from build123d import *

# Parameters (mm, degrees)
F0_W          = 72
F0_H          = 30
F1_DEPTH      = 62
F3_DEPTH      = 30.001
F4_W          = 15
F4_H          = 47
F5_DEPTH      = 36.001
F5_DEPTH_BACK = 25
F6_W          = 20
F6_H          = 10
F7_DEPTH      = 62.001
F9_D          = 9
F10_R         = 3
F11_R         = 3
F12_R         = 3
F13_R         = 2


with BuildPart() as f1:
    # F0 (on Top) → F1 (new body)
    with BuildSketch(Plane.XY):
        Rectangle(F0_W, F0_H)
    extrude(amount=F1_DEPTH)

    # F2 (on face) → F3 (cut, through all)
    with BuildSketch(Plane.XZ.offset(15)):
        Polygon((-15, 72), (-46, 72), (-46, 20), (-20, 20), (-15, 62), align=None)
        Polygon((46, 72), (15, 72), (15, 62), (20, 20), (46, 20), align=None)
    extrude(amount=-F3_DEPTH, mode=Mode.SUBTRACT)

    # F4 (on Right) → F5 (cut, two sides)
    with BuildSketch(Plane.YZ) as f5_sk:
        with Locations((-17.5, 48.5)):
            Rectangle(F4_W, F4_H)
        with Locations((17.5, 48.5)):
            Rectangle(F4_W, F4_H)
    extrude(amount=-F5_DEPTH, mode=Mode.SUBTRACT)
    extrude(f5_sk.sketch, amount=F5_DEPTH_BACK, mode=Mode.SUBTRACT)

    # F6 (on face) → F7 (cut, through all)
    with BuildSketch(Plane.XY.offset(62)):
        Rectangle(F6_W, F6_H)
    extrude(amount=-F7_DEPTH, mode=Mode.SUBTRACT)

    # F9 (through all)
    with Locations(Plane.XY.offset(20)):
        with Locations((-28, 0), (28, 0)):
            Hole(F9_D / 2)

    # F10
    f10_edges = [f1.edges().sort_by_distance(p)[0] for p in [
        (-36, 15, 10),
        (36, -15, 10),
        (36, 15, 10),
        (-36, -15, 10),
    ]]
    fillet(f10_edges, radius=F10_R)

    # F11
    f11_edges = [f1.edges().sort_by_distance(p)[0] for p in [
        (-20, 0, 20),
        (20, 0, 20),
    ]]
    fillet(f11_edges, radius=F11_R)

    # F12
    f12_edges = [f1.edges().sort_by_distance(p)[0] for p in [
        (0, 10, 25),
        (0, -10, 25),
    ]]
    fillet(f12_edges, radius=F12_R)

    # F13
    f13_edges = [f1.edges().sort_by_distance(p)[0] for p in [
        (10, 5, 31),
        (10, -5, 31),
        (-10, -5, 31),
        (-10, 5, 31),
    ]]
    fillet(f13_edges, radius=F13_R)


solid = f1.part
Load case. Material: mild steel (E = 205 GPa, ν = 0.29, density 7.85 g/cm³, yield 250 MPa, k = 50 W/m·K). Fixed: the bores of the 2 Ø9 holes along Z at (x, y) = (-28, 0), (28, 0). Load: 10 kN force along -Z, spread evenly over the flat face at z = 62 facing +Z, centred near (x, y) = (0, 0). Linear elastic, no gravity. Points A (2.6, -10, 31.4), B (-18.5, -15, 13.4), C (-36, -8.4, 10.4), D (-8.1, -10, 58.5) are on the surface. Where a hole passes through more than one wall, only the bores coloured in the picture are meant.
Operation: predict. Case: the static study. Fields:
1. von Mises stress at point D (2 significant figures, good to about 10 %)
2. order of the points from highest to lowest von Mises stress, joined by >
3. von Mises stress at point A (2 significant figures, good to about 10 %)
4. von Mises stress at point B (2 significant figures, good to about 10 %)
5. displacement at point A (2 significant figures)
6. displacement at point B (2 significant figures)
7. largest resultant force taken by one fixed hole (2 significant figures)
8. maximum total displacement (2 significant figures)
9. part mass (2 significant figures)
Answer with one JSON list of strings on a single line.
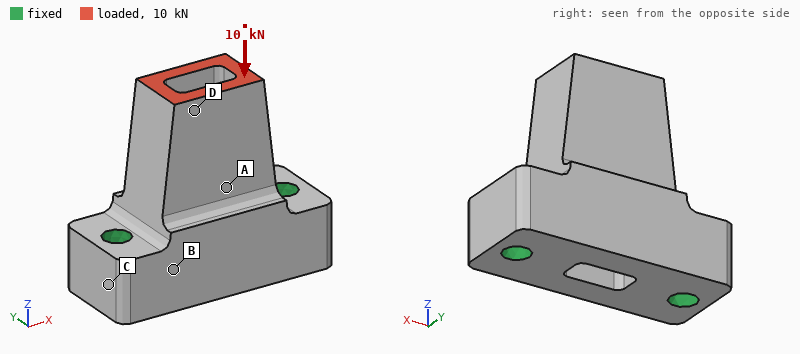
["24 MPa", "D > A > B > C", "17 MPa", "11 MPa", "3.1 µm", "1.5 µm", "5.2 kN", "6.3 µm", "470 g"]
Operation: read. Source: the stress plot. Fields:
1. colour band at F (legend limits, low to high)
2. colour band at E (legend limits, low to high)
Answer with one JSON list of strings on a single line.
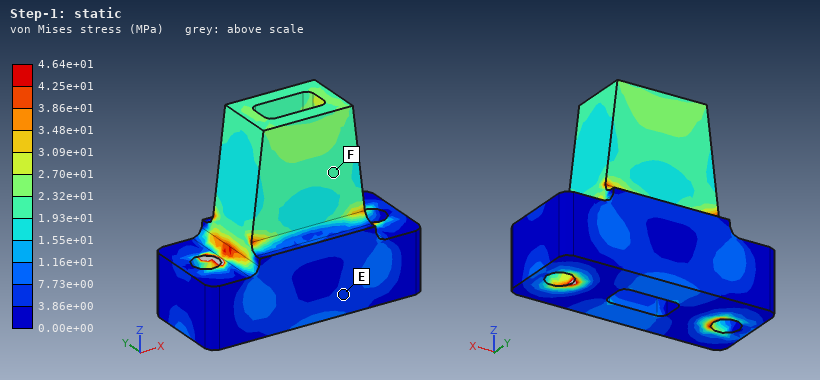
["1.93e+01 to 2.32e+01 MPa", "3.86e+00 to 7.73e+00 MPa"]
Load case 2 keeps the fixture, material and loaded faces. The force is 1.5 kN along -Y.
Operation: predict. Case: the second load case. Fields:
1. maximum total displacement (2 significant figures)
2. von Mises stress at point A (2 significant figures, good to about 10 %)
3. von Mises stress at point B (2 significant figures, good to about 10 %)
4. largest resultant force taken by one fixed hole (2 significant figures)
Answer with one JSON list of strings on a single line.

["20 µm", "19 MPa", "17 MPa", "750 N"]
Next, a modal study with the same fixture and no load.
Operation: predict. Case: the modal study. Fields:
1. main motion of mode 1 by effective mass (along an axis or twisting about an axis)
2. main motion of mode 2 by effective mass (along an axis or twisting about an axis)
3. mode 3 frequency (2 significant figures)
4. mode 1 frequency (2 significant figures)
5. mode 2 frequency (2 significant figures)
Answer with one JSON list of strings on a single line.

["along Y", "along X", "16 kHz", "6500 Hz", "12 kHz"]
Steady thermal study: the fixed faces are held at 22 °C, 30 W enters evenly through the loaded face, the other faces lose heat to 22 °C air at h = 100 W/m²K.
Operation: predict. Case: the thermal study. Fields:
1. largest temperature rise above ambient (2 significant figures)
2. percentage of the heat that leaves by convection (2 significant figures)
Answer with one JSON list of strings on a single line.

["42 K", "50 %"]
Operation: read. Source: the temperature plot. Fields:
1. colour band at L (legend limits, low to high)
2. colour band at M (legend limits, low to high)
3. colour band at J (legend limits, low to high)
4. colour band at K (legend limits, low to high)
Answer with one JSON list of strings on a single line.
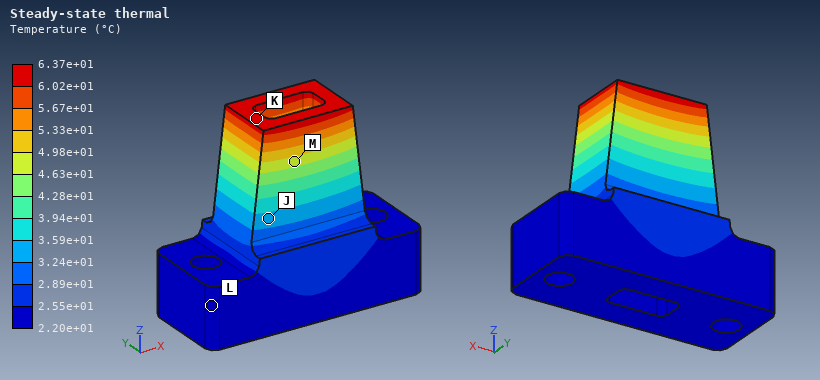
["2.20e+01 to 2.55e+01 °C", "4.63e+01 to 4.98e+01 °C", "3.24e+01 to 3.59e+01 °C", "6.02e+01 to 6.37e+01 °C"]
